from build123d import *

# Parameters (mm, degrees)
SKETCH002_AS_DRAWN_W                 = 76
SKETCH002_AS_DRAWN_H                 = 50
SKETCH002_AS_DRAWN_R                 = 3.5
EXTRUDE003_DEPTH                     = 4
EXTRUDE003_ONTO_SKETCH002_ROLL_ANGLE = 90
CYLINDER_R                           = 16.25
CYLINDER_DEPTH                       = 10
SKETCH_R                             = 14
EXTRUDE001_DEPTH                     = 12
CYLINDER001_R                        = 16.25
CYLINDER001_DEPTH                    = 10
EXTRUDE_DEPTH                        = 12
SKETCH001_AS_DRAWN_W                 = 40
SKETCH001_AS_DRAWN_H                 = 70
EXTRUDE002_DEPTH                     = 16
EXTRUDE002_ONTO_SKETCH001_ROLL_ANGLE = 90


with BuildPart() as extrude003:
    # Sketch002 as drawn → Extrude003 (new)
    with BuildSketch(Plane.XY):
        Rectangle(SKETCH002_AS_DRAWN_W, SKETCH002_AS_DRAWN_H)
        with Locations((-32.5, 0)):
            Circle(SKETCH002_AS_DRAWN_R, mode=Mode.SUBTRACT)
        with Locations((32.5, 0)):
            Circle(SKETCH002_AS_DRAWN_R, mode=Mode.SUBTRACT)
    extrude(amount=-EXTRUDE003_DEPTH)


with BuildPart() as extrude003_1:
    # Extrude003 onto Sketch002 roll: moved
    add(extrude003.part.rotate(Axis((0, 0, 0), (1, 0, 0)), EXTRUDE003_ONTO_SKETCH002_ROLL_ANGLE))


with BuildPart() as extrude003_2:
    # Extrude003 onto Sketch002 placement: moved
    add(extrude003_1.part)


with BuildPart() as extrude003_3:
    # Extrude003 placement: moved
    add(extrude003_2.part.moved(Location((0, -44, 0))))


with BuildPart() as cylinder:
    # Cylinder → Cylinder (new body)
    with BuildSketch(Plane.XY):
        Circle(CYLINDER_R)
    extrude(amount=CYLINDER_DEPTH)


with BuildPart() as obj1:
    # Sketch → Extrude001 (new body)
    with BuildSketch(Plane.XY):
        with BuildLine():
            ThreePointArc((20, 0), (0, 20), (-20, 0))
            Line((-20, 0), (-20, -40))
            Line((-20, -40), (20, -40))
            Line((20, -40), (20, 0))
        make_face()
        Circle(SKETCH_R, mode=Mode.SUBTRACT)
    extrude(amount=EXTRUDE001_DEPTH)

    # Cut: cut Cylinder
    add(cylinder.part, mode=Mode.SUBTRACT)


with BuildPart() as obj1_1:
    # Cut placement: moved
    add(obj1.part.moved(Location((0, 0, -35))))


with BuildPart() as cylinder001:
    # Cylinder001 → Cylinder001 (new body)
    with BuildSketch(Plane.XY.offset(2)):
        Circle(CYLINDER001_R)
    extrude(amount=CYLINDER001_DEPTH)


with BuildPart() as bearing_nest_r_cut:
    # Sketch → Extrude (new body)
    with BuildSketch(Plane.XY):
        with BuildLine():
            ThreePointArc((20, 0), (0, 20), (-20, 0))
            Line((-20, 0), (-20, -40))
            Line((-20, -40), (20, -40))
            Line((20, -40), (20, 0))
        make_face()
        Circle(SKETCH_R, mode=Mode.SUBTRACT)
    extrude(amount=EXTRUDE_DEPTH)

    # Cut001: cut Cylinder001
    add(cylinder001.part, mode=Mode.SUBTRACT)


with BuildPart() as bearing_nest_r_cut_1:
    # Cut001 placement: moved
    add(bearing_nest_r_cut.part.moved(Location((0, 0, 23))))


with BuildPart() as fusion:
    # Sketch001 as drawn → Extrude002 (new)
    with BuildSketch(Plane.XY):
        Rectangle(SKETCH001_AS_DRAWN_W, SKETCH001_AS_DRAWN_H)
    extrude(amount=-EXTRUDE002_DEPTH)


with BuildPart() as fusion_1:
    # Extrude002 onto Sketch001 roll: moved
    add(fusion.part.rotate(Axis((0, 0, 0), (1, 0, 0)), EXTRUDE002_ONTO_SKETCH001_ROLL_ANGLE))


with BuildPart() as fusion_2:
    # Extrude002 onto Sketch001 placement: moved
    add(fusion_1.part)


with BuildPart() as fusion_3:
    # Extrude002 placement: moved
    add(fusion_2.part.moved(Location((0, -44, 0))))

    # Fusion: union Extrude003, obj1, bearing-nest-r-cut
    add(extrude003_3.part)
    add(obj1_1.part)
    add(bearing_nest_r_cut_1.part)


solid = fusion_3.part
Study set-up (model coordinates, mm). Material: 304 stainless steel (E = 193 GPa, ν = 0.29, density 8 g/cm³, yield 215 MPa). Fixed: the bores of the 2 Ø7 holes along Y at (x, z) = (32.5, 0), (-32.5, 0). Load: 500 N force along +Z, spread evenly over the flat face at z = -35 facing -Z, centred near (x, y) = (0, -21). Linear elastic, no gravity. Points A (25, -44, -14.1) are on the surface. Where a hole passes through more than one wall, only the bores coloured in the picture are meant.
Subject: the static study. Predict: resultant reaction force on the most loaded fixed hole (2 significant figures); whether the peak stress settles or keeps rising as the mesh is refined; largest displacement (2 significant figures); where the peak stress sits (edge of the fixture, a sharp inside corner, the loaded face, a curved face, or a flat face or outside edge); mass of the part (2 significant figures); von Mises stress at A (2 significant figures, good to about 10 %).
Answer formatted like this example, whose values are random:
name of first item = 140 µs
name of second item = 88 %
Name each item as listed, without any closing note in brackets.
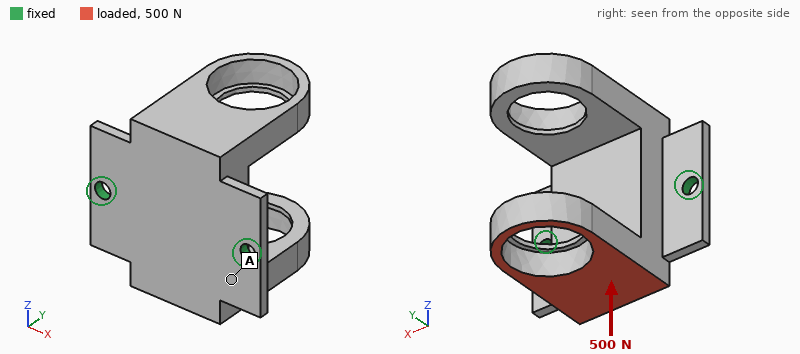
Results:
resultant reaction force on the most loaded fixed hole = 250 N
whether the peak stress settles or keeps rising as the mesh is refined = keeps rising
largest displacement = 66 µm
where the peak stress sits = edge of the fixture
mass of the part = 600 g
von Mises stress at A = 8.7 MPa
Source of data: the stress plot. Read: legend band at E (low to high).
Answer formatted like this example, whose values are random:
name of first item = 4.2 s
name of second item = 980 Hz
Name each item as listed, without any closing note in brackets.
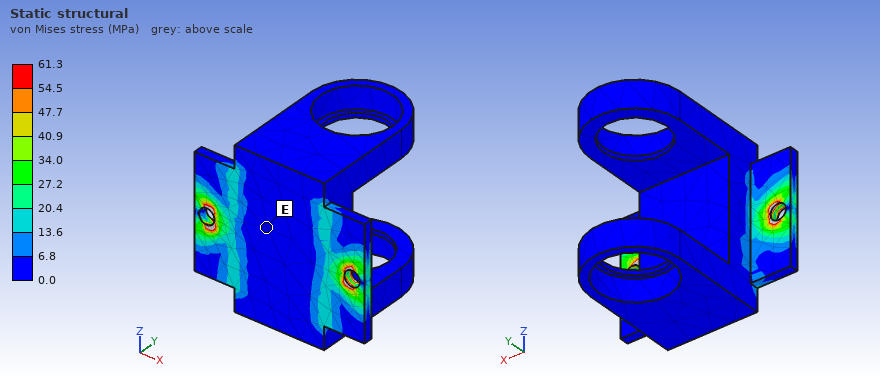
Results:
legend band at E = 0.0 to 6.8 MPa
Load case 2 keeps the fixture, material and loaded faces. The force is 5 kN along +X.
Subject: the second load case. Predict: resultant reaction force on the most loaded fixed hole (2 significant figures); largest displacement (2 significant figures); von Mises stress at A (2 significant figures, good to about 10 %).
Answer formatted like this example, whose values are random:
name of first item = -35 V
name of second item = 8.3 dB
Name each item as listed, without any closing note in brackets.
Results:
resultant reaction force on the most loaded fixed hole = 4.2 kN
largest displacement = 0.10 mm
von Mises stress at A = 29 MPa
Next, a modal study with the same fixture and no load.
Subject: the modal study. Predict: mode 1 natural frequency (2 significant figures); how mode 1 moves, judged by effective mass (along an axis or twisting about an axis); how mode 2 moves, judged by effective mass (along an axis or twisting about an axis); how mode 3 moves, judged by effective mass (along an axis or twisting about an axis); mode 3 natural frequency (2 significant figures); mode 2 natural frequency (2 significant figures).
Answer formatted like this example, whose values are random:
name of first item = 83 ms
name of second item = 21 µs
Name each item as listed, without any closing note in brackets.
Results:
mode 1 natural frequency = 780 Hz
how mode 1 moves, judged by effective mass = along Z
how mode 2 moves, judged by effective mass = along Y
how mode 3 moves, judged by effective mass = along X
mode 3 natural frequency = 2900 Hz
mode 2 natural frequency = 2800 Hz
